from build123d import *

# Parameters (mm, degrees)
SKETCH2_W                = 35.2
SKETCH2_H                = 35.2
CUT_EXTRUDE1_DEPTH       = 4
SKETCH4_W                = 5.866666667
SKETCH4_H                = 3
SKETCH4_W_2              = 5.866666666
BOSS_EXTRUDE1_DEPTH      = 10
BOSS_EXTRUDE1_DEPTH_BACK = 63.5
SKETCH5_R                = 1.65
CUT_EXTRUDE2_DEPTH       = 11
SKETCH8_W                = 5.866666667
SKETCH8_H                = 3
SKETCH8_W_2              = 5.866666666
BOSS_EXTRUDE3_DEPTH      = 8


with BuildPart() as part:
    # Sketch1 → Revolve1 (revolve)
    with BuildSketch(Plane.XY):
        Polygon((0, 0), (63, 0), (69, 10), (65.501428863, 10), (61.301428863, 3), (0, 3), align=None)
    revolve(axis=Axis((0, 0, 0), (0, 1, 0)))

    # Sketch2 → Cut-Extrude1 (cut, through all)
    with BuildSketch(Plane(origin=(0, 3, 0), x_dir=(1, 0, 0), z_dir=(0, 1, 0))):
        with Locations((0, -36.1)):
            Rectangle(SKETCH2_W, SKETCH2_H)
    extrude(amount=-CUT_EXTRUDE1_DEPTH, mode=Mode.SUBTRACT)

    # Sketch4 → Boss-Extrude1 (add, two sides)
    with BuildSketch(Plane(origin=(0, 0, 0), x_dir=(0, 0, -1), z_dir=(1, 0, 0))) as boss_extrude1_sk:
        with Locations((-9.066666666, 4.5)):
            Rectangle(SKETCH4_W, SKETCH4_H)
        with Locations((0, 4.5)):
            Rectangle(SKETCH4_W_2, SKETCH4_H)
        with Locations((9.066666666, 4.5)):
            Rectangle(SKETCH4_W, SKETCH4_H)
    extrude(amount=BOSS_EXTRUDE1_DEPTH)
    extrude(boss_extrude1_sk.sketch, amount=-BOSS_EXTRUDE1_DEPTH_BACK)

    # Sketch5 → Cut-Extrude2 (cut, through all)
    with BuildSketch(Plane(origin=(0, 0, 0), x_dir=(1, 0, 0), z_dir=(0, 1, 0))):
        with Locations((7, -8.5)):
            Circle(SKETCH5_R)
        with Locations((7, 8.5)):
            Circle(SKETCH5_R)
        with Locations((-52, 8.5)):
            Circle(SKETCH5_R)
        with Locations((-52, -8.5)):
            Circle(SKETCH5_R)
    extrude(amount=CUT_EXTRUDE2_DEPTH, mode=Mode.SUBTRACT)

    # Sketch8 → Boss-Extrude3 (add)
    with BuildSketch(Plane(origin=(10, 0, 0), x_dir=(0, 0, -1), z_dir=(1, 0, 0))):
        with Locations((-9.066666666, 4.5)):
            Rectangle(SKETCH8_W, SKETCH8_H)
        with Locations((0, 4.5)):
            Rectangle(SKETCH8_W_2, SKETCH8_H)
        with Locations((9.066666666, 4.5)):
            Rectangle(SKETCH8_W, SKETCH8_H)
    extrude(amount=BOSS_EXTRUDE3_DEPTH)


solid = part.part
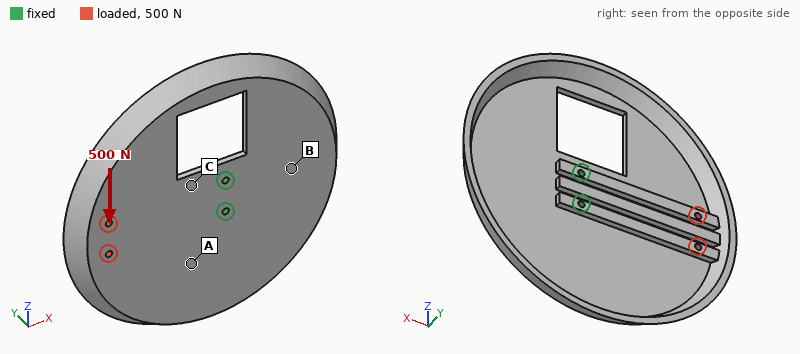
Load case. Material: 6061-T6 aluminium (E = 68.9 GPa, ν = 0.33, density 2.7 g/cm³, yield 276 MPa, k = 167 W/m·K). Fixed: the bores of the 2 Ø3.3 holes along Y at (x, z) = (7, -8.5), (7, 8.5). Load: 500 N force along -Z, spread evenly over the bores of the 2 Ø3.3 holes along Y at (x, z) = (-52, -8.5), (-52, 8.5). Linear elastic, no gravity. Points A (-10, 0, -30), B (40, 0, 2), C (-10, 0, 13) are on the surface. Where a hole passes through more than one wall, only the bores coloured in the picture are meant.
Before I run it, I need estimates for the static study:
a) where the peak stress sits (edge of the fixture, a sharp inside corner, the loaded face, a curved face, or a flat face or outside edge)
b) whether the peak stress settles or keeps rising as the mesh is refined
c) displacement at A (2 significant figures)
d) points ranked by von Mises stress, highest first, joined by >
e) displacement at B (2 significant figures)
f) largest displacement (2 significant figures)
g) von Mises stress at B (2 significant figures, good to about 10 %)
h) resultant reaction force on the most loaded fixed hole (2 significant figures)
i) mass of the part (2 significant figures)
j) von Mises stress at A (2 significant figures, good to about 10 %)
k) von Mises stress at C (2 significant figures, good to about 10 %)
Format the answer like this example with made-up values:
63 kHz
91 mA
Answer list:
edge of the fixture
keeps rising
19 µm
C > B > A
14 µm
52 µm
4.1 MPa
1.5 kN
130 g
2.0 MPa
8.1 MPa
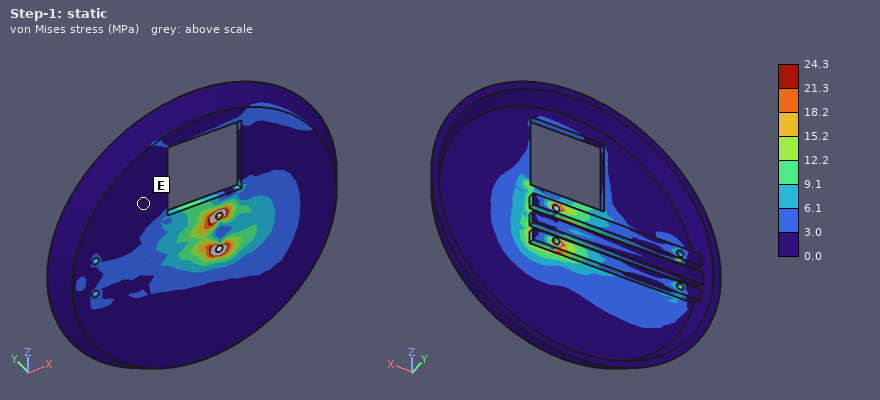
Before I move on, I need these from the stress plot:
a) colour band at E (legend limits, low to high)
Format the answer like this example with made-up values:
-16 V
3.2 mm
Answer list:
0.0 to 3.0 MPa
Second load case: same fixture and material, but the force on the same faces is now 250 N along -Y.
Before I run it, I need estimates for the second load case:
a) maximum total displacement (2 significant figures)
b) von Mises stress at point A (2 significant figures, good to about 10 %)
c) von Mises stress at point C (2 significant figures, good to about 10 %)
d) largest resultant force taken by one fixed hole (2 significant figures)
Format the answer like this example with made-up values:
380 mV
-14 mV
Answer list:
0.56 mm
18 MPa
40 MPa
180 N
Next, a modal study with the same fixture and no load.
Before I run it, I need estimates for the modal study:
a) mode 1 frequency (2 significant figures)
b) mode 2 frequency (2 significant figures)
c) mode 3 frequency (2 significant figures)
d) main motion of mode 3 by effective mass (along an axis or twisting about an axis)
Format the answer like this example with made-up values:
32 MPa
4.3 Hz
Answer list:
590 Hz
630 Hz
910 Hz
along Y
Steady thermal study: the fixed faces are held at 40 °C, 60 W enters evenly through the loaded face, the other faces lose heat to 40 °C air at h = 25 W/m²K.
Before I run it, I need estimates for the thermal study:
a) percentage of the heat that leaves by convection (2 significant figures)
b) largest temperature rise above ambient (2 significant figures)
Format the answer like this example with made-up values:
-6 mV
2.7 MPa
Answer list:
35 %
78 K
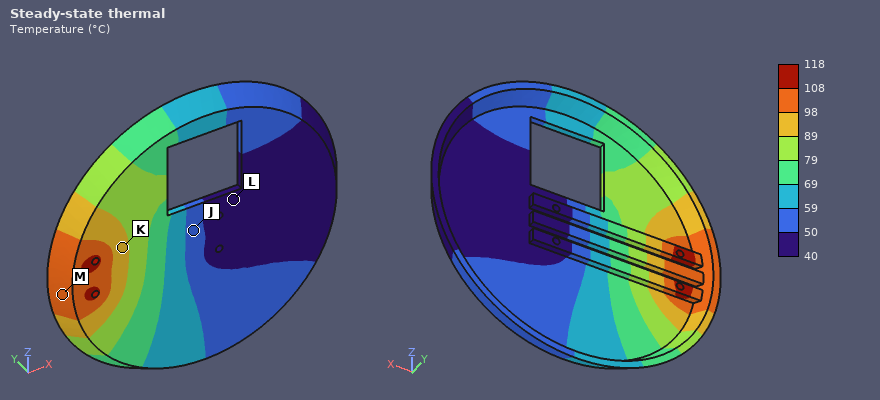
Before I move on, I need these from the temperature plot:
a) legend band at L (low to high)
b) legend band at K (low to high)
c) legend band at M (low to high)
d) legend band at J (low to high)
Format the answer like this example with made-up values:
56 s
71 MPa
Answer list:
40 to 50 °C
89 to 98 °C
98 to 108 °C
50 to 59 °C
